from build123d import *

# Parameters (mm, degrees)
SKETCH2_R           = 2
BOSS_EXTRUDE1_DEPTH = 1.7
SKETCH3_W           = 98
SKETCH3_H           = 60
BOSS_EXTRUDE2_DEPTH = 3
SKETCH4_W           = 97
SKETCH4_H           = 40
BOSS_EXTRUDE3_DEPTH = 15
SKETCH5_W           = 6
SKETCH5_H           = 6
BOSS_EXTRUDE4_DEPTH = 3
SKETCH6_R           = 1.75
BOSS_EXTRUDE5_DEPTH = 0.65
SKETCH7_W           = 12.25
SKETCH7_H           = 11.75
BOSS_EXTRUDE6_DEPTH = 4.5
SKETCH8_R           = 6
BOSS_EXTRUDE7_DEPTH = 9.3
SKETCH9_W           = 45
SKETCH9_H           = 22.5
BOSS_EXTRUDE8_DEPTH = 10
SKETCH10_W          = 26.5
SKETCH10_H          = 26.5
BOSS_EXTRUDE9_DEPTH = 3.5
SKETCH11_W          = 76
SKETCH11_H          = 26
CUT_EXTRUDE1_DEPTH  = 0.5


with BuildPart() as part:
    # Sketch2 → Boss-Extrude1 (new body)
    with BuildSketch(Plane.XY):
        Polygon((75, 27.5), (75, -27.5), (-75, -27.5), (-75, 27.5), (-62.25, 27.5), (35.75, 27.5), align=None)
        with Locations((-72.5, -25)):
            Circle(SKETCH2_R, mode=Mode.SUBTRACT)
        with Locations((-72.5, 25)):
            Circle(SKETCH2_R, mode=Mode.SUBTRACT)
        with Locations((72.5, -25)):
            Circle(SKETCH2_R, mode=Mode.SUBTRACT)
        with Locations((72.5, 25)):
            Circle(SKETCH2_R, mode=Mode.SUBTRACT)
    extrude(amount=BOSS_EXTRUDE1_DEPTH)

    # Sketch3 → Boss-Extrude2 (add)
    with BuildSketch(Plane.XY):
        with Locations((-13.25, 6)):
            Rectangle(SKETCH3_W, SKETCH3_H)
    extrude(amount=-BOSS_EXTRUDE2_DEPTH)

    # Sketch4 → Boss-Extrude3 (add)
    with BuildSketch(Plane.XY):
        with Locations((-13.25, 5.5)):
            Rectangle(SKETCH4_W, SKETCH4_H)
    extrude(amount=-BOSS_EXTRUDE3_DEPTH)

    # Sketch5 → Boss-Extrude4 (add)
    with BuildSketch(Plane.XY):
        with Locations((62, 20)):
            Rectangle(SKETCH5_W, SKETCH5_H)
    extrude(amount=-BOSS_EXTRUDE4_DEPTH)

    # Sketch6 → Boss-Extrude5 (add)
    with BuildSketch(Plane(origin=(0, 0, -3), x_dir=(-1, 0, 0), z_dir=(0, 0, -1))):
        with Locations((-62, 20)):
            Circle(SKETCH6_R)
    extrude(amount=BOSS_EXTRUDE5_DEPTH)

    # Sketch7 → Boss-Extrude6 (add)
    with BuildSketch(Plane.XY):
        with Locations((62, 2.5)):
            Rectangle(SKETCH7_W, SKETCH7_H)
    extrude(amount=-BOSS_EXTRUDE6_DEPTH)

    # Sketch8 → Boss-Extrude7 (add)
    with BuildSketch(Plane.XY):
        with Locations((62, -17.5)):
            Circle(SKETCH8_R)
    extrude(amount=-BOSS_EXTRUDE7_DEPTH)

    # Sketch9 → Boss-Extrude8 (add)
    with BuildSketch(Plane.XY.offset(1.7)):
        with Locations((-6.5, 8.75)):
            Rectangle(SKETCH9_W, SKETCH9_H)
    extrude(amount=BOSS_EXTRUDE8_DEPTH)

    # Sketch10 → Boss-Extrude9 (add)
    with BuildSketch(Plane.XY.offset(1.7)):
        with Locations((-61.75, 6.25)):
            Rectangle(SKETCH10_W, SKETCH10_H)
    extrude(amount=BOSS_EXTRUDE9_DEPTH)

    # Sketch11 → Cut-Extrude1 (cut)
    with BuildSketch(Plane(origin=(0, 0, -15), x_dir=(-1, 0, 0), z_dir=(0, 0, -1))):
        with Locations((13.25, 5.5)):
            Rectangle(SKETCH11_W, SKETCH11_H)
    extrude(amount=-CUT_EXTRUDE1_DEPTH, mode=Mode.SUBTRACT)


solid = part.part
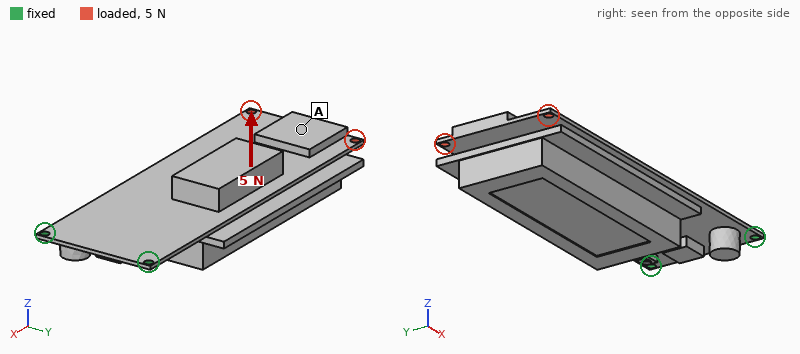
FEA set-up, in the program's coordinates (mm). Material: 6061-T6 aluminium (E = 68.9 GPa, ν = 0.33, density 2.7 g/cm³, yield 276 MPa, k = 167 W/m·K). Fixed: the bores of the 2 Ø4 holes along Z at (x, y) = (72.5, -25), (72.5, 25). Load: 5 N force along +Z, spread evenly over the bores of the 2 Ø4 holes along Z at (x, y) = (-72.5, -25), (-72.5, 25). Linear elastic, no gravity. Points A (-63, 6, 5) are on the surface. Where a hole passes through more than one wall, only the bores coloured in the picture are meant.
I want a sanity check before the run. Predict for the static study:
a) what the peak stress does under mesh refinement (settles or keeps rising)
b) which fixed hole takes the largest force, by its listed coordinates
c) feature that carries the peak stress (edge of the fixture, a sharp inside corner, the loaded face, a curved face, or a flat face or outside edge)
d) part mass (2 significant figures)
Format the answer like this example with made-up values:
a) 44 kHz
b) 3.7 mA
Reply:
a) keeps rising
b) (72.5, 25)
c) edge of the fixture
d) 250 g
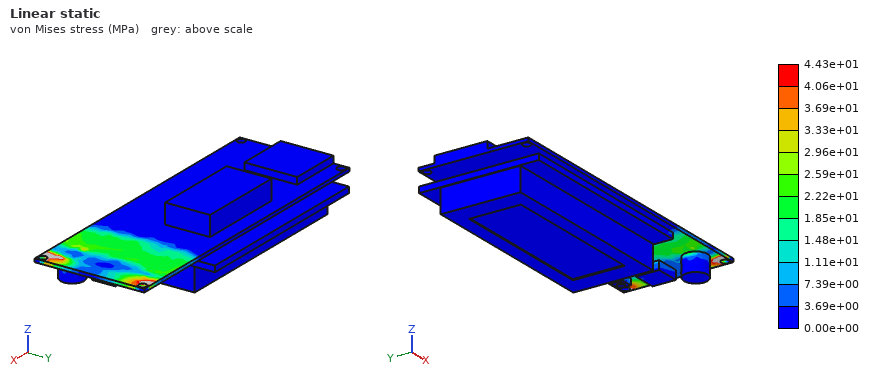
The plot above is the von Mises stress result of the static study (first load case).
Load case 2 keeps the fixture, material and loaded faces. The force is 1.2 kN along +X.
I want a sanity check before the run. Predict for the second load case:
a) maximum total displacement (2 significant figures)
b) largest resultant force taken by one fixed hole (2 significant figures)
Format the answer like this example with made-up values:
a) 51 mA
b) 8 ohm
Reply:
a) 0.14 mm
b) 640 N
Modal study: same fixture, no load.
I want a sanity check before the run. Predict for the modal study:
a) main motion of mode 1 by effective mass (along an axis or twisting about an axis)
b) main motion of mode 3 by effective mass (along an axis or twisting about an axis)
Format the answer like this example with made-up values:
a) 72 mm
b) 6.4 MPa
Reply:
a) along Z
b) along Z
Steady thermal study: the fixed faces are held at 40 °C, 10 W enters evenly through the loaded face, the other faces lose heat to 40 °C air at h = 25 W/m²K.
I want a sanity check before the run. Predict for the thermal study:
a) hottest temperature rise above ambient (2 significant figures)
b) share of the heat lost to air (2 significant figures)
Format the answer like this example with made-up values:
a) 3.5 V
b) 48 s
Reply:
a) 45 K
b) 70 %
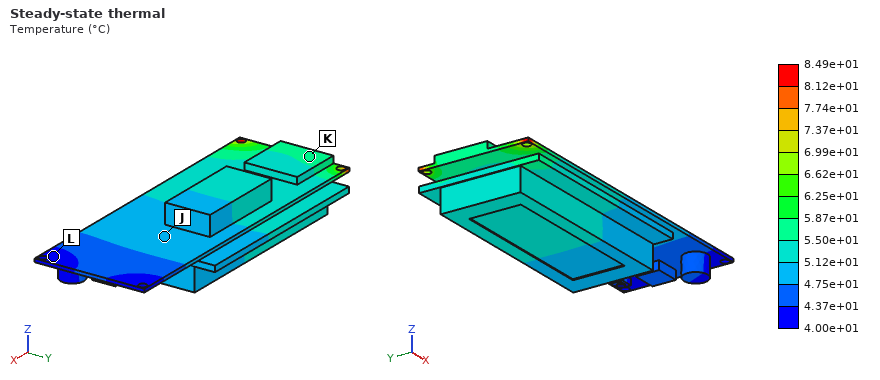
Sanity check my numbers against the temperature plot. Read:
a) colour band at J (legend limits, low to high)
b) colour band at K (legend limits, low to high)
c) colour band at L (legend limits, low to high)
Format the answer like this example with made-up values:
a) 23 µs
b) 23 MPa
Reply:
a) 4.75e+01 to 5.12e+01 °C
b) 5.50e+01 to 5.87e+01 °C
c) 4.00e+01 to 4.37e+01 °C
